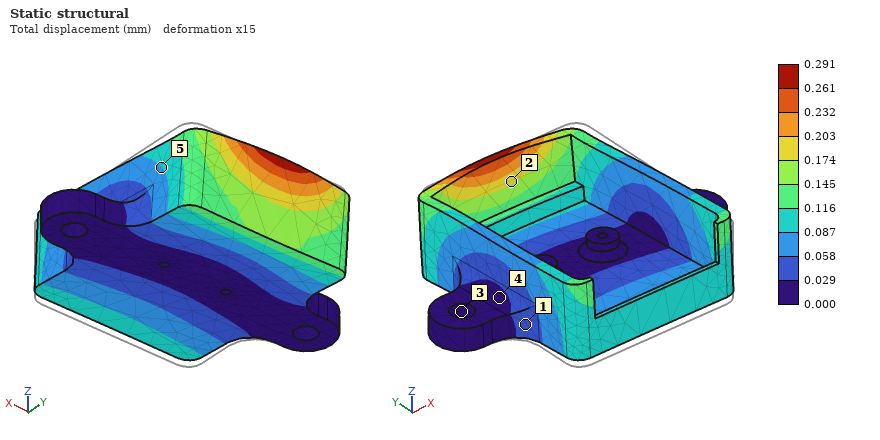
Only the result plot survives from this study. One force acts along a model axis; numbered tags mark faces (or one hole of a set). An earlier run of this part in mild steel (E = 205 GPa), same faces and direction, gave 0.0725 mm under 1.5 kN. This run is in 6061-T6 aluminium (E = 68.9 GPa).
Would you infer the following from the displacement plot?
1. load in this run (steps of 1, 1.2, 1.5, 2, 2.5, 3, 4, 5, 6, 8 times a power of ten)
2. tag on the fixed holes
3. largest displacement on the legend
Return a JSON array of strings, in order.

["2 kN", "3", "0.291 mm"]
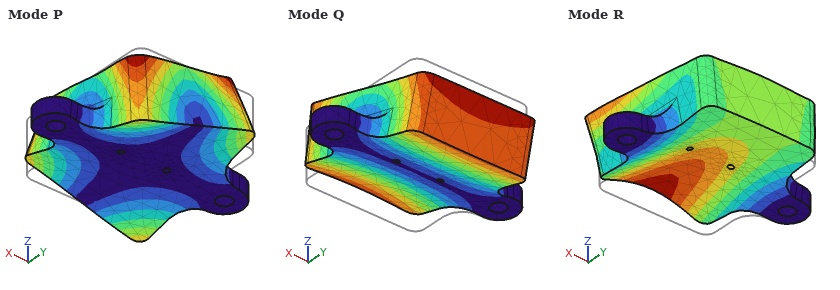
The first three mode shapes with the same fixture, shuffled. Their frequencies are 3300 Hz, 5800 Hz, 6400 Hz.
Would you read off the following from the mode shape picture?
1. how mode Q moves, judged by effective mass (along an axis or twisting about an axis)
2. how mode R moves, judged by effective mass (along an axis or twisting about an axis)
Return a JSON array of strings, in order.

["twisting about X", "along Z"]
